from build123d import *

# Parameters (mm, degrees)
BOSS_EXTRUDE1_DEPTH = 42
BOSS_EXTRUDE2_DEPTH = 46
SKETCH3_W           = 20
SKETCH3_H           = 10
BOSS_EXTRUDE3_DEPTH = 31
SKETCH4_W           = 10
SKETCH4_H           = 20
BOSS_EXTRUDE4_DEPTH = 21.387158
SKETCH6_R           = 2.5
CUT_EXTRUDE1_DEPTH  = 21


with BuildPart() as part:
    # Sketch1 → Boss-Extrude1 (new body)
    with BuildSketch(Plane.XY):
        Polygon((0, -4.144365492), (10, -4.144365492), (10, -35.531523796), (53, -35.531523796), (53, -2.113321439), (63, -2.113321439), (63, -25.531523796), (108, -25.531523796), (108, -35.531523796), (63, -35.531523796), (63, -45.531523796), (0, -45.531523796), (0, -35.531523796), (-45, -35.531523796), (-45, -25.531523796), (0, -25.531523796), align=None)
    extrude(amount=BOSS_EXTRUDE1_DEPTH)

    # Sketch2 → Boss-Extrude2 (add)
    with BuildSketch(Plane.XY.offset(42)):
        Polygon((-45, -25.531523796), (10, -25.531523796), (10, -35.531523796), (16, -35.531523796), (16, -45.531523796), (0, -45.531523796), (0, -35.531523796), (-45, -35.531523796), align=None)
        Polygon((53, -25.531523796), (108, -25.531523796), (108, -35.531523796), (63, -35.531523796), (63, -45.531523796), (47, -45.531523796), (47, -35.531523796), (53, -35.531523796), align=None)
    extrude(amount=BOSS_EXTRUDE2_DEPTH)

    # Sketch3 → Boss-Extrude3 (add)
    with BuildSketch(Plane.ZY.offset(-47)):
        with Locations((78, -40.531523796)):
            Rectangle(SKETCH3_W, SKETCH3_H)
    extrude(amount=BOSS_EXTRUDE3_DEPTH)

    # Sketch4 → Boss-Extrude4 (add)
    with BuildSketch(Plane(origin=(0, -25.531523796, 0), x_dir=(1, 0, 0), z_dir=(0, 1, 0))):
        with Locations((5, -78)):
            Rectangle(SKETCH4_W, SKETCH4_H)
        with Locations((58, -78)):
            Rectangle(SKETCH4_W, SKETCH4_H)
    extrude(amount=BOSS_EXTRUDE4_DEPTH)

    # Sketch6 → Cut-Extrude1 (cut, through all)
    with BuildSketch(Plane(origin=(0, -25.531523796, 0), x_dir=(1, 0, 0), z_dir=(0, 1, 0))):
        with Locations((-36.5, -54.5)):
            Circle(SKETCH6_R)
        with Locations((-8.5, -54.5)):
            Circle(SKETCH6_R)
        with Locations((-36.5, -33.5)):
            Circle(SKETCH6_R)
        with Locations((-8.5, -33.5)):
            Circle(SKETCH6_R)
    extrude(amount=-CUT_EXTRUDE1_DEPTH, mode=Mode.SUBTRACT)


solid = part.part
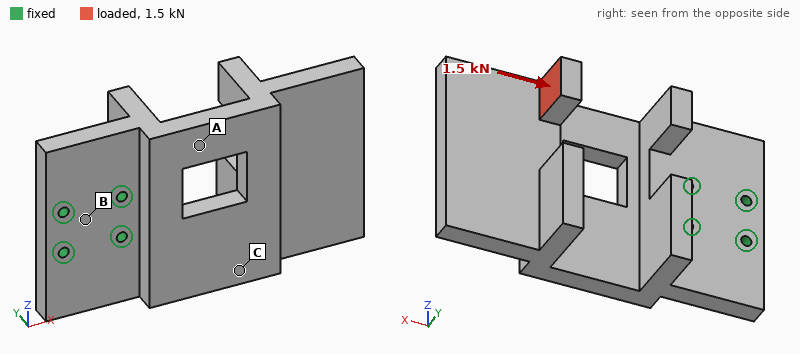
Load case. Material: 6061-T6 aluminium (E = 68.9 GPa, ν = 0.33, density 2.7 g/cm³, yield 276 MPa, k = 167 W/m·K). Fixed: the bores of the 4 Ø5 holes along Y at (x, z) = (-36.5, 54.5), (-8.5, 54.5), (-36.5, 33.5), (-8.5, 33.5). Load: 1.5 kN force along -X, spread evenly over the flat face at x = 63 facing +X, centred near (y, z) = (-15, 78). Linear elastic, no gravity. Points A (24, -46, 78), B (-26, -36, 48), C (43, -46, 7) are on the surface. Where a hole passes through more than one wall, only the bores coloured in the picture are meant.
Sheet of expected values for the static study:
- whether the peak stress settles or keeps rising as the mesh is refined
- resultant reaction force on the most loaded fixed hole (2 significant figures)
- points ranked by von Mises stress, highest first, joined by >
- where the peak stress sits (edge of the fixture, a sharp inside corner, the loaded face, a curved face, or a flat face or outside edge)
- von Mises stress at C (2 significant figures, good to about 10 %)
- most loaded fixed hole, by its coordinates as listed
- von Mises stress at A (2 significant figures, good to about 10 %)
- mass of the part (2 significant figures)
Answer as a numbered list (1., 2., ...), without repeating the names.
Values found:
1. keeps rising
2. 1.3 kN
3. A > C > B
4. edge of the fixture
5. 29 MPa
6. (-8.5, 54.5)
7. 38 MPa
8. 460 g
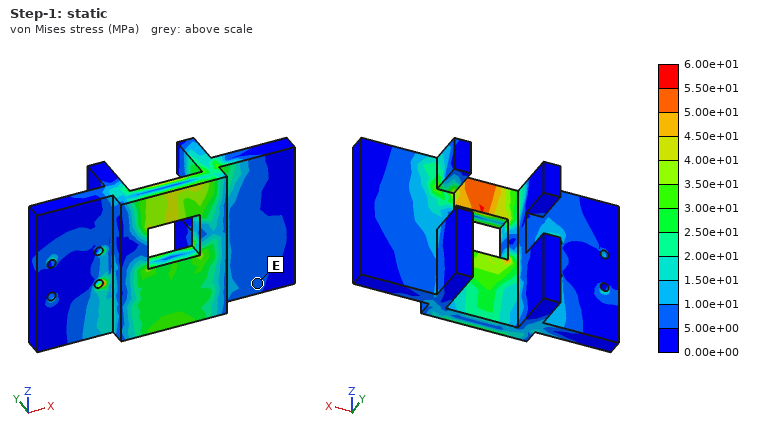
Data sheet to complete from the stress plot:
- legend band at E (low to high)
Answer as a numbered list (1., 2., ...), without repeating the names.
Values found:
1. 5.00e+00 to 1.00e+01 MPa
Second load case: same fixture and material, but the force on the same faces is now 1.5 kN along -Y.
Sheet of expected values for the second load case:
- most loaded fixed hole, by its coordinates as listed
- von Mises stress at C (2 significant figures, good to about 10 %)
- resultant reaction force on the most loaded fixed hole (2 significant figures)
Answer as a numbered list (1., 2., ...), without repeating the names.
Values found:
1. (-8.5, 54.5)
2. 41 MPa
3. 3.2 kN
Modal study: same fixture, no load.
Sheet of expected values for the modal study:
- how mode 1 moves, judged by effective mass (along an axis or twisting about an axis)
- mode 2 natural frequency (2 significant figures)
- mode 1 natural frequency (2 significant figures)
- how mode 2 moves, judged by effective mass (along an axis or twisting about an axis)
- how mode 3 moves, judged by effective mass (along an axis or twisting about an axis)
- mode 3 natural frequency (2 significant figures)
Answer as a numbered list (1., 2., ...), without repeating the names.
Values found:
1. along Y
2. 1200 Hz
3. 470 Hz
4. along Z
5. along Z
6. 2000 Hz
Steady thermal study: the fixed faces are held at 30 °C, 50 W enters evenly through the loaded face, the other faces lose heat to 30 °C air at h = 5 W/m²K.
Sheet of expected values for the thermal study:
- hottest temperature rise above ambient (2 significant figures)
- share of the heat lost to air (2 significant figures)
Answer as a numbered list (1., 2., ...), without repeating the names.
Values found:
1. 66 K
2. 7.8 %
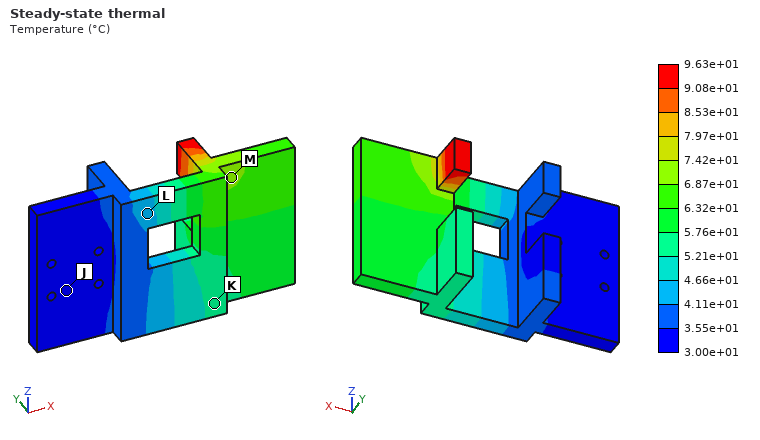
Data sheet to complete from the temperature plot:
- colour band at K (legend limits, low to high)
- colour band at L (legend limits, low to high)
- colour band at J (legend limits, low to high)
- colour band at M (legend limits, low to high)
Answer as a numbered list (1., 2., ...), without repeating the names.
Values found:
1. 5.21e+01 to 5.76e+01 °C
2. 4.11e+01 to 4.66e+01 °C
3. 3.00e+01 to 3.55e+01 °C
4. 6.87e+01 to 7.42e+01 °C
